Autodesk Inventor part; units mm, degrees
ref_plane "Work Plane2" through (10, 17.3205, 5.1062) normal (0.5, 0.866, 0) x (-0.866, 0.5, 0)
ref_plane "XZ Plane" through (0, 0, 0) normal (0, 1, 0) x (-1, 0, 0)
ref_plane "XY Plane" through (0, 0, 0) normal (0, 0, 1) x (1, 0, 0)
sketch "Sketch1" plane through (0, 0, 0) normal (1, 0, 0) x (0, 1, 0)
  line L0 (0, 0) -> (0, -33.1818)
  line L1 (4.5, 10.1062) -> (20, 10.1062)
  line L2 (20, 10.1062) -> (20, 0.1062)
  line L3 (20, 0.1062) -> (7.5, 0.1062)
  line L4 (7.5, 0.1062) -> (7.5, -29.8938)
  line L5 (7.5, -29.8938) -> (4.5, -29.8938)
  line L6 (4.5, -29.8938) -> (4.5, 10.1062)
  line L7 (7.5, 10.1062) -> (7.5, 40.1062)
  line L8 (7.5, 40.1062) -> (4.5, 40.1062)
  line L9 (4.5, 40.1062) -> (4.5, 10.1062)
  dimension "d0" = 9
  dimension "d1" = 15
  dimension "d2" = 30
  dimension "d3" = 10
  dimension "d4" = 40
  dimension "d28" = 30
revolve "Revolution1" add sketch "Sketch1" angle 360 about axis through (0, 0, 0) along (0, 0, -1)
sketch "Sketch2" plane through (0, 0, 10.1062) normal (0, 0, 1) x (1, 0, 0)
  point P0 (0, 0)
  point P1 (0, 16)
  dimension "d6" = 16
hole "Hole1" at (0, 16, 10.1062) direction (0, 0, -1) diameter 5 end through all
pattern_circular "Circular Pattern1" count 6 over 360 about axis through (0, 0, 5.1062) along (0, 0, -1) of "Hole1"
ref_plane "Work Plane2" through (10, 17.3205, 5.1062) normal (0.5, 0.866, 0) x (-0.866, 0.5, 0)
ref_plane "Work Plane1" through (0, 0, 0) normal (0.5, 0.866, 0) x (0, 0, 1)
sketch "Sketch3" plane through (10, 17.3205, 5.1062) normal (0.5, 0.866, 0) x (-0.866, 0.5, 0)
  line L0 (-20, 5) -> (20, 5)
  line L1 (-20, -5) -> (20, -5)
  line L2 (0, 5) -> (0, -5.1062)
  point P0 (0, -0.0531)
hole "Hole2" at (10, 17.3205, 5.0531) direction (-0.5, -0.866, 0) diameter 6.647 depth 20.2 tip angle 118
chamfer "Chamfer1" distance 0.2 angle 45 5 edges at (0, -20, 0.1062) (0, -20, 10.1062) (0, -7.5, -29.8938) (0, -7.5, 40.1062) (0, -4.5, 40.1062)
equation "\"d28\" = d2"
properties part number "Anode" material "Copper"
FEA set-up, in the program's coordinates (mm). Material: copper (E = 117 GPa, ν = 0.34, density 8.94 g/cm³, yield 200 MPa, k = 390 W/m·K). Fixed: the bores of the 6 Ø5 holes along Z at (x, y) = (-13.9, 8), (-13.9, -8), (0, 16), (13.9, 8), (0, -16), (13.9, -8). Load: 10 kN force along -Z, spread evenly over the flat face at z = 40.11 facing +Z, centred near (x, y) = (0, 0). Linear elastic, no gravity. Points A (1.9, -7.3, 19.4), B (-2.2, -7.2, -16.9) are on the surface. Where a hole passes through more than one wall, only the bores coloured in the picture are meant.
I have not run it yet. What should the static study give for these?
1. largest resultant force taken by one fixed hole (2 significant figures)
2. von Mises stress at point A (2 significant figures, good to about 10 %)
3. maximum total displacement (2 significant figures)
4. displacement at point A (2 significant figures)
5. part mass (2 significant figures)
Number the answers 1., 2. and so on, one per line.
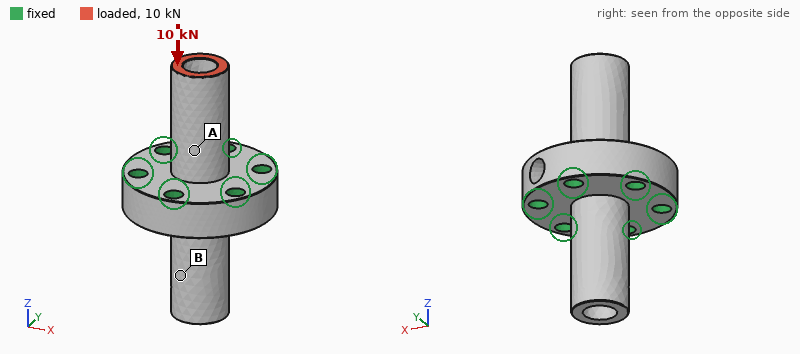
1. 1.8 kN
2. 85 MPa
3. 30 µm
4. 13 µm
5. 150 g
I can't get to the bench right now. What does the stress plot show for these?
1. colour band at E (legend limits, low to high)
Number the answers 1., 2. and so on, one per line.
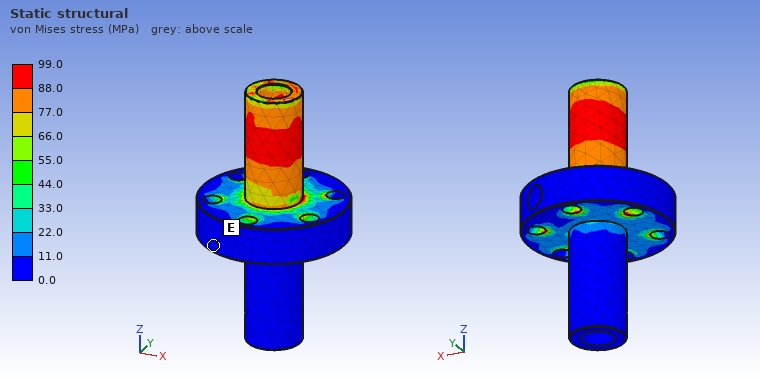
1. 0.0 to 11.0 MPa
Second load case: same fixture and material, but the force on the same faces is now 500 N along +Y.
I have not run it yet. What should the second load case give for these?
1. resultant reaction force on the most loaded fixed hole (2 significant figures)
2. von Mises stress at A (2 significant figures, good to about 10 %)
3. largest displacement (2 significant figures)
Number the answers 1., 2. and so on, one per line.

1. 510 N
2. 34 MPa
3. 33 µm
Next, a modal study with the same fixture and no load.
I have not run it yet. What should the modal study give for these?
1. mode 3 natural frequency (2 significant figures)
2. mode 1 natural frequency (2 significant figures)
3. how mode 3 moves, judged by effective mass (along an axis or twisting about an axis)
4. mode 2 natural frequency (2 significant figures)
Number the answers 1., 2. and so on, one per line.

1. 6900 Hz
2. 6200 Hz
3. along Y
4. 6200 Hz
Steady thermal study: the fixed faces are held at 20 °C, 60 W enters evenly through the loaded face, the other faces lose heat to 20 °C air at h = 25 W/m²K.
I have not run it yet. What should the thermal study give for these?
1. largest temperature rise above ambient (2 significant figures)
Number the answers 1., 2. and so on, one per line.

1. 45 K
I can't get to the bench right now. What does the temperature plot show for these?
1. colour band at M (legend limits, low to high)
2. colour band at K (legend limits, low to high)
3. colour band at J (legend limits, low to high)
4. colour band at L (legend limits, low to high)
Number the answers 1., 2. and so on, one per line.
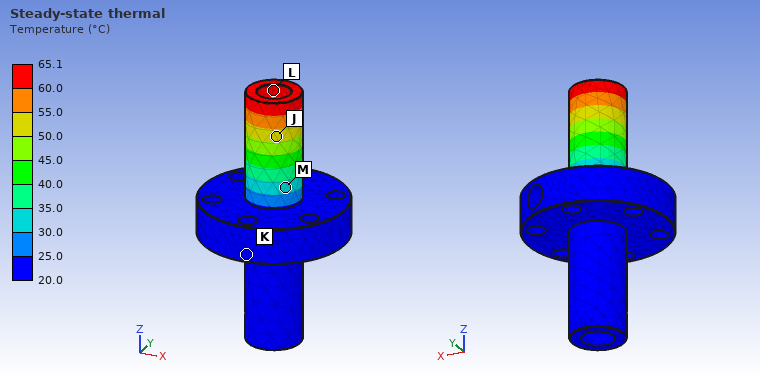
1. 30.0 to 35.0 °C
2. 20.0 to 25.0 °C
3. 50.0 to 55.0 °C
4. 60.0 to 65.1 °C
